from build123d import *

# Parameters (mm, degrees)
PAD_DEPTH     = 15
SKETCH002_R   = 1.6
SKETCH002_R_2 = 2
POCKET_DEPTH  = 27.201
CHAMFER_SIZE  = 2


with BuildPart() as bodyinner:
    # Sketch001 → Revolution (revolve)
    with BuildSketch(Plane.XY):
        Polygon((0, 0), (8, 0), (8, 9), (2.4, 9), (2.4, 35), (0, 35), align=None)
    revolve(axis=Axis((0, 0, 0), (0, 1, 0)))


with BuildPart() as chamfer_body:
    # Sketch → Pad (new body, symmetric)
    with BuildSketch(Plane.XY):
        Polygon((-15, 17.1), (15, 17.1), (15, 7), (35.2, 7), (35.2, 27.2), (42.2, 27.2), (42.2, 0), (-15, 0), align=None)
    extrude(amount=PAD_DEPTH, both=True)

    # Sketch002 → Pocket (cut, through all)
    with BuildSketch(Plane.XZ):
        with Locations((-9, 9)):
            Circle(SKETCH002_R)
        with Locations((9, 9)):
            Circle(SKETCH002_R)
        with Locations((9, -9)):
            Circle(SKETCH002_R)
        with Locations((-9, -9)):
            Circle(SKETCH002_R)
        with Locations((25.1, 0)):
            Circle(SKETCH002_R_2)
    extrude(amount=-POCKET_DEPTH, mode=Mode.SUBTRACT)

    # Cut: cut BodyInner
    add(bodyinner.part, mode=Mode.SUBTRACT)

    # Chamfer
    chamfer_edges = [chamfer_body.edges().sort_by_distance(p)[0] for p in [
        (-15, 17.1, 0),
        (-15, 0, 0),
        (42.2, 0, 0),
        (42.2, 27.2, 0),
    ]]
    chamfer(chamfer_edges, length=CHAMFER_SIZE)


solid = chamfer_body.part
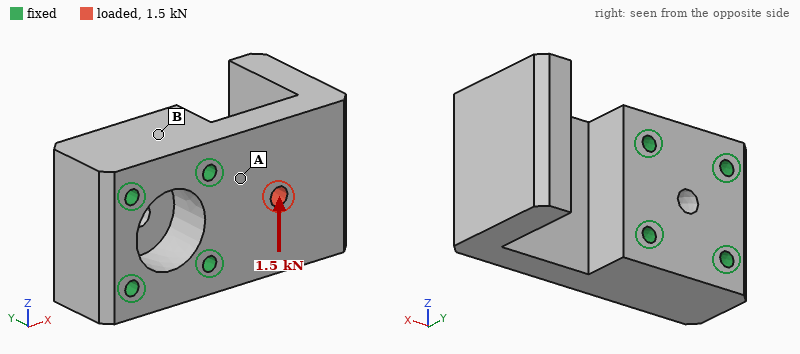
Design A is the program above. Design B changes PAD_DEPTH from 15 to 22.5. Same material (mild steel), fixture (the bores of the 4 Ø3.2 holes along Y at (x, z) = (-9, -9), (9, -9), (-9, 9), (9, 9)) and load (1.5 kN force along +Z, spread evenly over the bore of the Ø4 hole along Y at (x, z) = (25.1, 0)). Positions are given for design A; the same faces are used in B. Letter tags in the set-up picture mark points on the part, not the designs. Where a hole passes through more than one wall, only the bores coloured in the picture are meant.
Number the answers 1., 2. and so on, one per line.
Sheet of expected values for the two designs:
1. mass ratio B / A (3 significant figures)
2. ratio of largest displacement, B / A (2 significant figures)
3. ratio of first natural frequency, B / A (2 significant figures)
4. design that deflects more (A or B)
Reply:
1. 1.56
2. 0.61
3. 1.0
4. A
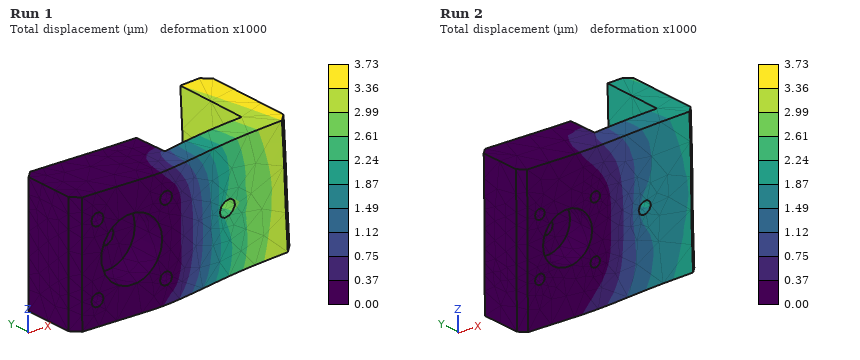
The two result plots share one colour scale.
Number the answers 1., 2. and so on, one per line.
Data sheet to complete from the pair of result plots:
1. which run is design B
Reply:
1. Run 2
